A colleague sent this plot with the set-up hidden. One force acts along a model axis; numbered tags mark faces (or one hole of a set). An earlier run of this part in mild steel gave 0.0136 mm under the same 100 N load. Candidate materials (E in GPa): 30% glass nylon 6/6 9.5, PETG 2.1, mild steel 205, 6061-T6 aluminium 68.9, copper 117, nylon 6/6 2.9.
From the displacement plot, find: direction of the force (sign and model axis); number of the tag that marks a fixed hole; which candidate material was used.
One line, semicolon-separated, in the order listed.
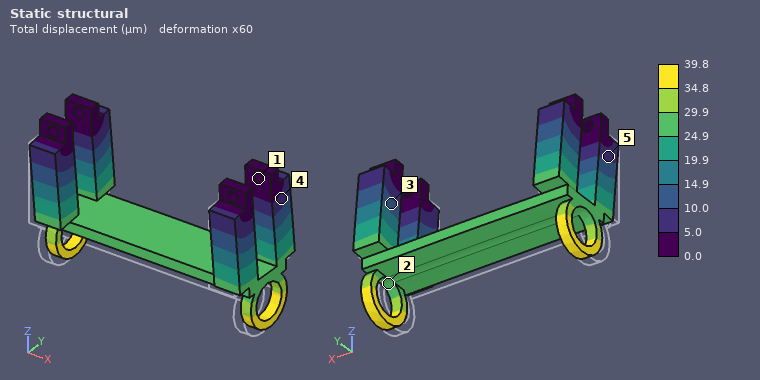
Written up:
+Y; 1; 6061-T6 aluminium
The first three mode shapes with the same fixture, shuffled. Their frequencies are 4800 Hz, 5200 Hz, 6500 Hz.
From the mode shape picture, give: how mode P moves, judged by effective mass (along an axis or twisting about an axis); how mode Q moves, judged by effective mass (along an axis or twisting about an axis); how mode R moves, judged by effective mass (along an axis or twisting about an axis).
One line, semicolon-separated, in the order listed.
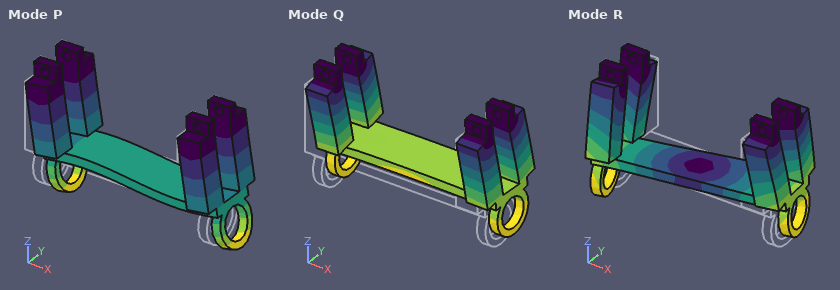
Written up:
along X; along Y; twisting about Z
